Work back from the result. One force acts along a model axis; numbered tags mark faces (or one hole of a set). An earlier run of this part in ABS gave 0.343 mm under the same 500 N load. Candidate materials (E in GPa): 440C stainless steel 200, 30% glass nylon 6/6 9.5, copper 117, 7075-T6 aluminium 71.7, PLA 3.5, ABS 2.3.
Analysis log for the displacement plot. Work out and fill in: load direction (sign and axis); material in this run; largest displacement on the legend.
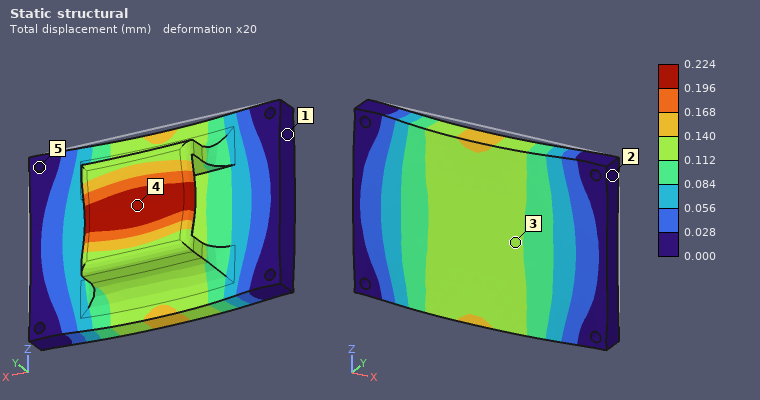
-Y
PLA
0.224 mm
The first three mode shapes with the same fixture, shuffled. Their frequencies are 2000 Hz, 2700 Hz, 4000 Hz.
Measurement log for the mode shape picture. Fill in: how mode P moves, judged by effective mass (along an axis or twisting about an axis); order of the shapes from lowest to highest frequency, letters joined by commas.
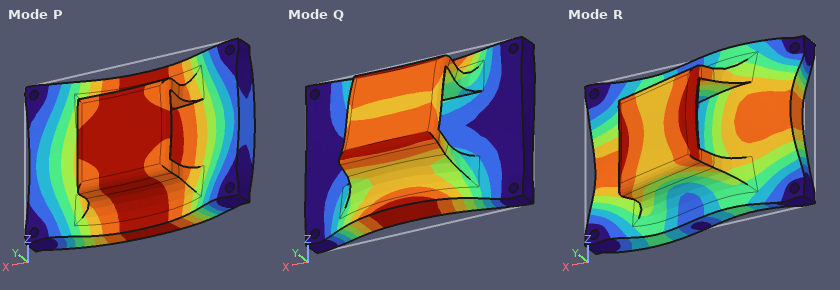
along Y
P, Q, R
